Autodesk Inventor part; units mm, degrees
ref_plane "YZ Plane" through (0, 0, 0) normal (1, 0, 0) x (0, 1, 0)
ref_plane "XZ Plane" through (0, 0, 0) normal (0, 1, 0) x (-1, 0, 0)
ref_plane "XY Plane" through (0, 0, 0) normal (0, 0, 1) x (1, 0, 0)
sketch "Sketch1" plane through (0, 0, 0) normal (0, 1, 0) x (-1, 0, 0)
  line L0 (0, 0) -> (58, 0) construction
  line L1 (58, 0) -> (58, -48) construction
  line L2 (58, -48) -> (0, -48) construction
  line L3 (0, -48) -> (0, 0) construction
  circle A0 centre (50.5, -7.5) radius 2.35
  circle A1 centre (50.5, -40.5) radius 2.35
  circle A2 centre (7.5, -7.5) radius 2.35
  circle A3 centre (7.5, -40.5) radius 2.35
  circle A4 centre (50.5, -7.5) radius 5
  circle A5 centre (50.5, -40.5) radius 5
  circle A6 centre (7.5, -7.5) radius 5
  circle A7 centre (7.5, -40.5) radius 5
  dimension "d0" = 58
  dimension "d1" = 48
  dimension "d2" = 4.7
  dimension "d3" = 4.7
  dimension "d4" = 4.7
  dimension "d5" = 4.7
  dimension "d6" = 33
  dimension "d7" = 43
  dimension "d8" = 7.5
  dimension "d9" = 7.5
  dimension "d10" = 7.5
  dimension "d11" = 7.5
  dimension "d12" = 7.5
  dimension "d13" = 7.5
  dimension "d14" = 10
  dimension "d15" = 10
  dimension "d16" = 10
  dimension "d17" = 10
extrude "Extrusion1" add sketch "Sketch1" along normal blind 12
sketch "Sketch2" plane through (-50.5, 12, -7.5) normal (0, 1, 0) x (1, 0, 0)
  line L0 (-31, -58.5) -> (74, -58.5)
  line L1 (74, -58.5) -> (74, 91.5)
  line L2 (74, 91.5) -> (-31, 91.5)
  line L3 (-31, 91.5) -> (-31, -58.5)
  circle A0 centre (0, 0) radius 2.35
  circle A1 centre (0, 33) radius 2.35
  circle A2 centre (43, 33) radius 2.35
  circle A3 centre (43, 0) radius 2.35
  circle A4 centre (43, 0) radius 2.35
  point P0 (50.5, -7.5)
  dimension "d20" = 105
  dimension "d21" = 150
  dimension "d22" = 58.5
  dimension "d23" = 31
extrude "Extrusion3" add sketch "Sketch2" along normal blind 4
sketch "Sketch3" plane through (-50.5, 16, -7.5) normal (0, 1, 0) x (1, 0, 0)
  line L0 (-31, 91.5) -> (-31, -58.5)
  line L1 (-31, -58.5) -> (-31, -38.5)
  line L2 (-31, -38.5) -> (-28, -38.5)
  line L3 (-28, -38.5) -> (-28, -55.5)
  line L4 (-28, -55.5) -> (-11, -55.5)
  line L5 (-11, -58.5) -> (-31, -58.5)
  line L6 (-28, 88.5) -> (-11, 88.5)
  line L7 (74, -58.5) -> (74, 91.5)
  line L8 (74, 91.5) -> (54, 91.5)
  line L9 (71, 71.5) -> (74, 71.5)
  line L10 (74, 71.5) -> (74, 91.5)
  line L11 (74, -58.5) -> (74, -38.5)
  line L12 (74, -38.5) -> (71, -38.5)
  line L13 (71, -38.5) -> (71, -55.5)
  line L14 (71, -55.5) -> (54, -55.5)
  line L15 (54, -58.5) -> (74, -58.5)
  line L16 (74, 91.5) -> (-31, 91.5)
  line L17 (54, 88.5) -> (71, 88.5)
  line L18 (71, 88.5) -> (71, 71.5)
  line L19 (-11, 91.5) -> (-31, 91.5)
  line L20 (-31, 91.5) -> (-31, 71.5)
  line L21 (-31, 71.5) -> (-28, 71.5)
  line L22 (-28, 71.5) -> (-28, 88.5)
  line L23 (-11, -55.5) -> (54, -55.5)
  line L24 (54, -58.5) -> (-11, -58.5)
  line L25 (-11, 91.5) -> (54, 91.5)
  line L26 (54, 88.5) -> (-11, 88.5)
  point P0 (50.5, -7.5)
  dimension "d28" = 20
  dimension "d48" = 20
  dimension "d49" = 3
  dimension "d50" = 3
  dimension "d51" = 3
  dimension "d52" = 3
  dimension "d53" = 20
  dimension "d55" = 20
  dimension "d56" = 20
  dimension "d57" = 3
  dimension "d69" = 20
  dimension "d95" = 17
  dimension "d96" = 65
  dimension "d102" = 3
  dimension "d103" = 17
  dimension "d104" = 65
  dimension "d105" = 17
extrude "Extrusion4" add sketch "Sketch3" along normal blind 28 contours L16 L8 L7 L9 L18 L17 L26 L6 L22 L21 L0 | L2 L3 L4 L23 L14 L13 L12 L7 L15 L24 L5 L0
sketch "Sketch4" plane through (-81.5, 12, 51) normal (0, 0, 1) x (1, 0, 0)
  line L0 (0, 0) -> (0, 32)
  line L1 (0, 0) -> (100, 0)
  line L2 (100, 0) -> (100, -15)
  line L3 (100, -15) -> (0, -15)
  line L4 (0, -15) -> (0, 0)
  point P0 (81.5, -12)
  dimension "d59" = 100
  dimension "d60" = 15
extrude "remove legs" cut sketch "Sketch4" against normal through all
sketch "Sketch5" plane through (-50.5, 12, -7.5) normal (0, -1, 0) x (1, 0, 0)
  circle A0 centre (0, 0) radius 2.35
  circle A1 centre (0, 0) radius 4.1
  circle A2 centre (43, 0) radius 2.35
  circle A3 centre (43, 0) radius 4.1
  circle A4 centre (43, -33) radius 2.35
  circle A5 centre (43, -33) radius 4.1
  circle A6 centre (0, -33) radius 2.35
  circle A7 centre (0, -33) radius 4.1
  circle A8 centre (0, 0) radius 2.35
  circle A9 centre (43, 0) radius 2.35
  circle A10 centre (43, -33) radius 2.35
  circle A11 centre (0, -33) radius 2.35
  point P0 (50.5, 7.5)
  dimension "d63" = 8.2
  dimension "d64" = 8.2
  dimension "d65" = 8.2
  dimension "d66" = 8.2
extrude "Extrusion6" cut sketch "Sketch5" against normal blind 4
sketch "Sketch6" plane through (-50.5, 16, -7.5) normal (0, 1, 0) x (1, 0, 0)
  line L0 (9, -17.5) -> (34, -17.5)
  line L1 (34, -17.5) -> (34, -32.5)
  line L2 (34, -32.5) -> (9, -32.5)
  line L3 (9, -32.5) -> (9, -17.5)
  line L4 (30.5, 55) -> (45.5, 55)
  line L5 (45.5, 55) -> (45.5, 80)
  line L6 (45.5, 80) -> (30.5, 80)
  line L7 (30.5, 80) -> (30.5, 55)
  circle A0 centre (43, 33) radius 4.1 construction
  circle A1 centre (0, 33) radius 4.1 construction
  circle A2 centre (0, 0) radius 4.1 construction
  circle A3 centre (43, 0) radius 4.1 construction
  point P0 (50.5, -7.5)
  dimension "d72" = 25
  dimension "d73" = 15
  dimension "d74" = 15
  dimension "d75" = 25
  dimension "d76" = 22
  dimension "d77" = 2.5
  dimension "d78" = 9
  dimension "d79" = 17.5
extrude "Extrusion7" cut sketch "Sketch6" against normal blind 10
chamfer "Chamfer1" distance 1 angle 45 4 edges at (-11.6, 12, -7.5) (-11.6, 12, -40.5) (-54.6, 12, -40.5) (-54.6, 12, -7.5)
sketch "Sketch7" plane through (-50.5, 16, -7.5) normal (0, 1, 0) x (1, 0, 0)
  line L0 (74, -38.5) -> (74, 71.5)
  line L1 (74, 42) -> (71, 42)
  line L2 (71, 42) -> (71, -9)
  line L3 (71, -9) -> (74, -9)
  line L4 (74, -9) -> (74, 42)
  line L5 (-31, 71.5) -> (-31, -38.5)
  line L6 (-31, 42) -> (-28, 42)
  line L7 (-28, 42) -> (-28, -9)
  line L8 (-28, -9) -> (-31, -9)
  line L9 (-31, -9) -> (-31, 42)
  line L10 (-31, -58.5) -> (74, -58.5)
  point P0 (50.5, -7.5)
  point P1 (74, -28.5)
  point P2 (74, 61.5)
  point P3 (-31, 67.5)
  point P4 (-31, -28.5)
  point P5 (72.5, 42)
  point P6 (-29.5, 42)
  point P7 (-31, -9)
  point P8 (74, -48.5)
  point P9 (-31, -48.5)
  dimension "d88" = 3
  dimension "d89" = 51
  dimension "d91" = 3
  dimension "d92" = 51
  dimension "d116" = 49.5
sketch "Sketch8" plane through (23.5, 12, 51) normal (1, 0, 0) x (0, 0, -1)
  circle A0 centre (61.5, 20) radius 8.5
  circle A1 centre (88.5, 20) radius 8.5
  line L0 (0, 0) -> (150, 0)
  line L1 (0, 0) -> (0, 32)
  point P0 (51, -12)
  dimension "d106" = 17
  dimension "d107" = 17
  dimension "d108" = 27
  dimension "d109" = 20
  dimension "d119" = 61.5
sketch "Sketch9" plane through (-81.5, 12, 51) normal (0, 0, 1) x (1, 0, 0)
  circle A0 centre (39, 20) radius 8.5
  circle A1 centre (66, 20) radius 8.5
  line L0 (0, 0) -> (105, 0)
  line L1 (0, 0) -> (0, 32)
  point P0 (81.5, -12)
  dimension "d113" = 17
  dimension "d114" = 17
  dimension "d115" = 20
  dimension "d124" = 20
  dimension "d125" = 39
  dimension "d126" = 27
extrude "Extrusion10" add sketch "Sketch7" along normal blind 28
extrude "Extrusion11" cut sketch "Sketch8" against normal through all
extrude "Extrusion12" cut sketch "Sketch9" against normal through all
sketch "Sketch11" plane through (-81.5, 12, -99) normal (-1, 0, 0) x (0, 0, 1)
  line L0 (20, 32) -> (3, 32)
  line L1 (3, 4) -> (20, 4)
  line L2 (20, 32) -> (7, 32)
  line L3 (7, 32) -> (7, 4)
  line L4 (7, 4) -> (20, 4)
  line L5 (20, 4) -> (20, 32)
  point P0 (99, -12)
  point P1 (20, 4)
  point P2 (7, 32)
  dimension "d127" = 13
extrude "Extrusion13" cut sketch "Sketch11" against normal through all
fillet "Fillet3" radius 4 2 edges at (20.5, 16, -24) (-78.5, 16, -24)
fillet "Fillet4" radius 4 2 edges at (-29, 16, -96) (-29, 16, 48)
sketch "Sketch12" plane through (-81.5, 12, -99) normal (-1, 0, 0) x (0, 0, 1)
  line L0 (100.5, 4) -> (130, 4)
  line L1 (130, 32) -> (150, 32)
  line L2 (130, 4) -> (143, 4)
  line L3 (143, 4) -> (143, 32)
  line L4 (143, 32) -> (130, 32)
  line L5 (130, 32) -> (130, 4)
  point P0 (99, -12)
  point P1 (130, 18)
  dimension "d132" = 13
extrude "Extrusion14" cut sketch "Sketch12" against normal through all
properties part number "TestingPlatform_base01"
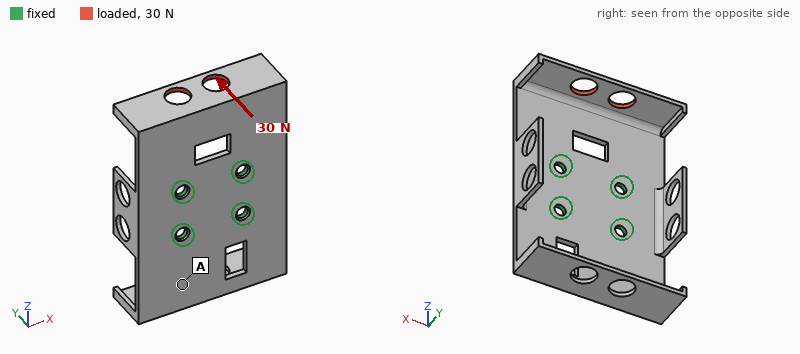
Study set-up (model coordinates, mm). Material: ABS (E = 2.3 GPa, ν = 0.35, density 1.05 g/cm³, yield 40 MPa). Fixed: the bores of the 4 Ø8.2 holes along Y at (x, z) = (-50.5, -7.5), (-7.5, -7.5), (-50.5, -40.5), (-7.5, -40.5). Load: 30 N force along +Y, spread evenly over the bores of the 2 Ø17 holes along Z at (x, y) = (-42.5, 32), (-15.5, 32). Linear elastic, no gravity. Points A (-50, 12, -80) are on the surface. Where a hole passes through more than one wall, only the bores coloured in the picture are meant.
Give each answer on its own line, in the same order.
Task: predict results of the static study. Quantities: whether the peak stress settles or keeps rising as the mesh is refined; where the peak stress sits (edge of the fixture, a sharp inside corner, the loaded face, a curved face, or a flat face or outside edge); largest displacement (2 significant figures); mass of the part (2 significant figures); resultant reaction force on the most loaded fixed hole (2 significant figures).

keeps rising
edge of the fixture
2.0 mm
86 g
25 N
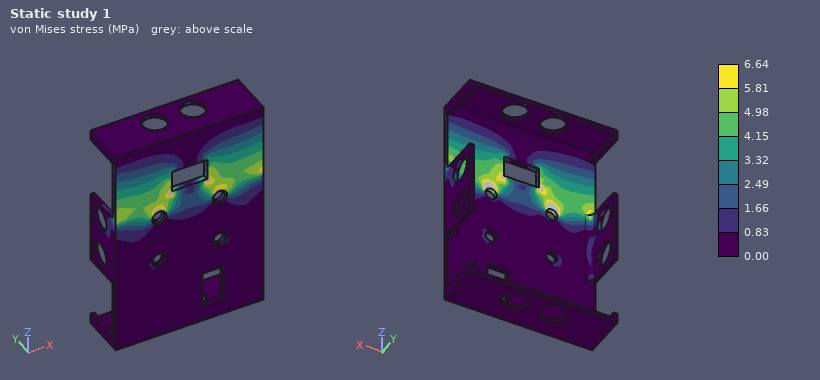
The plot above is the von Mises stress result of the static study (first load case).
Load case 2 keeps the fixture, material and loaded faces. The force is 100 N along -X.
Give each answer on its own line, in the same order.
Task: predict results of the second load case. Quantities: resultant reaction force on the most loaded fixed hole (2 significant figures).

92 N
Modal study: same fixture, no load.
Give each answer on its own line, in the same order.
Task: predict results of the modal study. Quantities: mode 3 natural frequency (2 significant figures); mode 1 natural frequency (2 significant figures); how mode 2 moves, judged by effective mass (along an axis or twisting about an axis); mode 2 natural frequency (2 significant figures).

260 Hz
170 Hz
along Y
180 Hz
